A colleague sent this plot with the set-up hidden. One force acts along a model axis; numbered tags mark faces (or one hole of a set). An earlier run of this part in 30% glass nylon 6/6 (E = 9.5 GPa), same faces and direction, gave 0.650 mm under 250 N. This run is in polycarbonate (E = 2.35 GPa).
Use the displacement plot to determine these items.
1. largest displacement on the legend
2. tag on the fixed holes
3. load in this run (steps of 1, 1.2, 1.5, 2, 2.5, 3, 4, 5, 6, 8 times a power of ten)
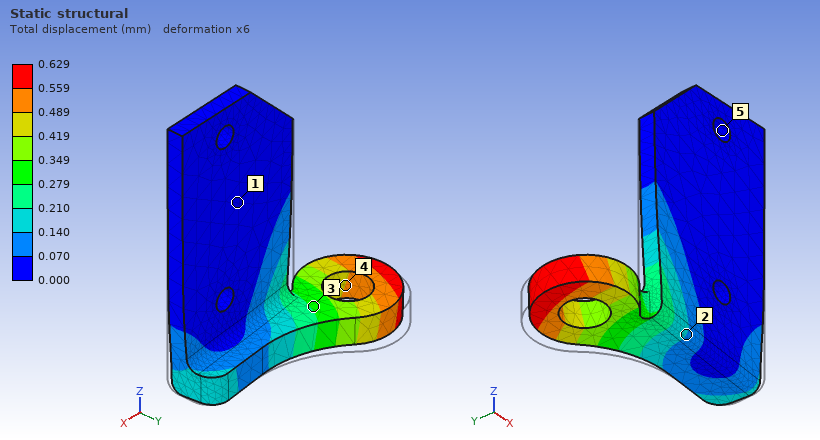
0.629 mm
5
60 N
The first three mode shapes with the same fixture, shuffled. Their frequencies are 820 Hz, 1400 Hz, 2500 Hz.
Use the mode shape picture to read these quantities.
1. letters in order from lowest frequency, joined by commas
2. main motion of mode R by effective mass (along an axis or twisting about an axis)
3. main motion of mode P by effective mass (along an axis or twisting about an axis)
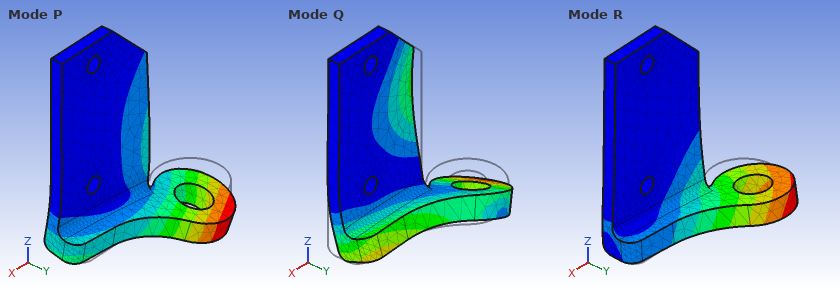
R, P, Q
along Y
along Z
